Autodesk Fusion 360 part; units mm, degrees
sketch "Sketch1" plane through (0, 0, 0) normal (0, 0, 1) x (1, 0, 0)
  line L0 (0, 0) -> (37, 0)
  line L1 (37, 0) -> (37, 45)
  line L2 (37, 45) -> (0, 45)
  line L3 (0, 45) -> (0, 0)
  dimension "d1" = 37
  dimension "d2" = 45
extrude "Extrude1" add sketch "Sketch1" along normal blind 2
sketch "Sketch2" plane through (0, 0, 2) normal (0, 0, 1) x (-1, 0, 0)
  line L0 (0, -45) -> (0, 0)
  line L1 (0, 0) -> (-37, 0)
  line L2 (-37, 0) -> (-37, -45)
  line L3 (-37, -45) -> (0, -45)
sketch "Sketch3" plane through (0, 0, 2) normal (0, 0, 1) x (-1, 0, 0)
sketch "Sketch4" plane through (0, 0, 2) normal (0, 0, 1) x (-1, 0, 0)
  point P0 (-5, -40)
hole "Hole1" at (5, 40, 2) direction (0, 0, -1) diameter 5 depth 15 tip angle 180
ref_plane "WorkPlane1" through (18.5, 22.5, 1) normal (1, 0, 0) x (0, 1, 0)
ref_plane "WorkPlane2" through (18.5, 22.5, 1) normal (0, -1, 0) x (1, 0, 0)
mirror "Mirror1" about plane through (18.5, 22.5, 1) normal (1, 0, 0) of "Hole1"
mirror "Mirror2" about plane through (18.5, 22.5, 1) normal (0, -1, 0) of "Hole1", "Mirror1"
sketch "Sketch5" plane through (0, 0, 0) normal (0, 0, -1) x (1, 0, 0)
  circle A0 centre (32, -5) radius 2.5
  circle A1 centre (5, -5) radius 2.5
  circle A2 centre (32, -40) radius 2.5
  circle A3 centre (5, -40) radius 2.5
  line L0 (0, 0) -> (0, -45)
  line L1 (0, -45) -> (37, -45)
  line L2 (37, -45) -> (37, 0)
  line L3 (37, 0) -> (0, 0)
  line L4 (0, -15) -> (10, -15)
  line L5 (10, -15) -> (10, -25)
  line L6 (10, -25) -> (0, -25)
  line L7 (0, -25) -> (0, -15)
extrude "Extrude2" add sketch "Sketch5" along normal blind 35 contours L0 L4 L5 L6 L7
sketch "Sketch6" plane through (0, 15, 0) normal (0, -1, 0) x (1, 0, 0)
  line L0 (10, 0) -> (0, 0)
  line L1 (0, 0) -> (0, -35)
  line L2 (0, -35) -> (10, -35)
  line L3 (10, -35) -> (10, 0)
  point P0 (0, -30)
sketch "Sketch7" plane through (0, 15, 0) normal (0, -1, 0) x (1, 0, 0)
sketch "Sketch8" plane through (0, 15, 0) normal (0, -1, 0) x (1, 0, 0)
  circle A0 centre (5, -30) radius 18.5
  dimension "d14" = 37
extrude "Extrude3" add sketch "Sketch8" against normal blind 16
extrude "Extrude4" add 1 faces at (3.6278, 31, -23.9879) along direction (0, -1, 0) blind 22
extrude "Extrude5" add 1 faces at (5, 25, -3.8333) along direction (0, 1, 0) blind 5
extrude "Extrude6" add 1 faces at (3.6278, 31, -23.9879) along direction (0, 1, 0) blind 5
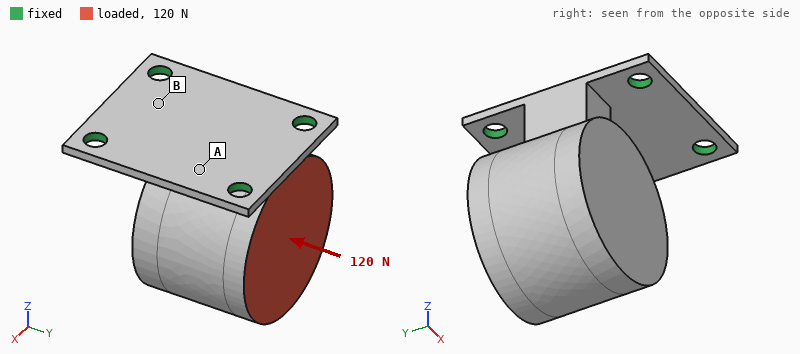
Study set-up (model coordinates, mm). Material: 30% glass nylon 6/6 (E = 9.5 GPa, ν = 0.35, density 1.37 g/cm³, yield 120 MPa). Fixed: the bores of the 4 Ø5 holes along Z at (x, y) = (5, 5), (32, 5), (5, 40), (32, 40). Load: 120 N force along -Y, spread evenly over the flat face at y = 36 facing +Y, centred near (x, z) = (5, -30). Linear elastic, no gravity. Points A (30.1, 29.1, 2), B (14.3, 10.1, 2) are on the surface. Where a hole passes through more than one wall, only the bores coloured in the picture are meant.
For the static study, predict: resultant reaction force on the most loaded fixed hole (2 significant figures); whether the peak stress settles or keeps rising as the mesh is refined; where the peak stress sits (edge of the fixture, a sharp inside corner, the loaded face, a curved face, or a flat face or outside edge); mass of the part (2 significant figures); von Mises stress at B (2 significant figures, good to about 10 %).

160 N
keeps rising
edge of the fixture
47 g
12 MPa
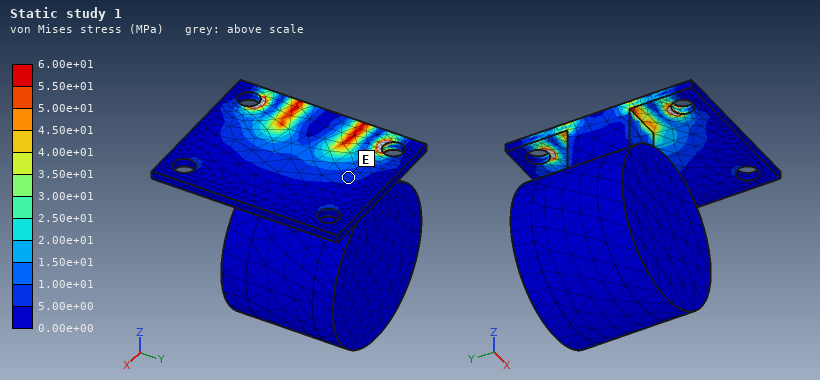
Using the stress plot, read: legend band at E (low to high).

5.00e+00 to 1.00e+01 MPa
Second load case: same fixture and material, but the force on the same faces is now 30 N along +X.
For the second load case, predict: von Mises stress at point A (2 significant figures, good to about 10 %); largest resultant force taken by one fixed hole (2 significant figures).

3.1 MPa
24 N
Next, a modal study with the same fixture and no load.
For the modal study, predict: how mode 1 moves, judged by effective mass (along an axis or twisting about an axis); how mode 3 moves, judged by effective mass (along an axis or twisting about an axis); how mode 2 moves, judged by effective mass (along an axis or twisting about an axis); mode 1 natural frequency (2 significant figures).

along X
along Z
along Y
190 Hz
